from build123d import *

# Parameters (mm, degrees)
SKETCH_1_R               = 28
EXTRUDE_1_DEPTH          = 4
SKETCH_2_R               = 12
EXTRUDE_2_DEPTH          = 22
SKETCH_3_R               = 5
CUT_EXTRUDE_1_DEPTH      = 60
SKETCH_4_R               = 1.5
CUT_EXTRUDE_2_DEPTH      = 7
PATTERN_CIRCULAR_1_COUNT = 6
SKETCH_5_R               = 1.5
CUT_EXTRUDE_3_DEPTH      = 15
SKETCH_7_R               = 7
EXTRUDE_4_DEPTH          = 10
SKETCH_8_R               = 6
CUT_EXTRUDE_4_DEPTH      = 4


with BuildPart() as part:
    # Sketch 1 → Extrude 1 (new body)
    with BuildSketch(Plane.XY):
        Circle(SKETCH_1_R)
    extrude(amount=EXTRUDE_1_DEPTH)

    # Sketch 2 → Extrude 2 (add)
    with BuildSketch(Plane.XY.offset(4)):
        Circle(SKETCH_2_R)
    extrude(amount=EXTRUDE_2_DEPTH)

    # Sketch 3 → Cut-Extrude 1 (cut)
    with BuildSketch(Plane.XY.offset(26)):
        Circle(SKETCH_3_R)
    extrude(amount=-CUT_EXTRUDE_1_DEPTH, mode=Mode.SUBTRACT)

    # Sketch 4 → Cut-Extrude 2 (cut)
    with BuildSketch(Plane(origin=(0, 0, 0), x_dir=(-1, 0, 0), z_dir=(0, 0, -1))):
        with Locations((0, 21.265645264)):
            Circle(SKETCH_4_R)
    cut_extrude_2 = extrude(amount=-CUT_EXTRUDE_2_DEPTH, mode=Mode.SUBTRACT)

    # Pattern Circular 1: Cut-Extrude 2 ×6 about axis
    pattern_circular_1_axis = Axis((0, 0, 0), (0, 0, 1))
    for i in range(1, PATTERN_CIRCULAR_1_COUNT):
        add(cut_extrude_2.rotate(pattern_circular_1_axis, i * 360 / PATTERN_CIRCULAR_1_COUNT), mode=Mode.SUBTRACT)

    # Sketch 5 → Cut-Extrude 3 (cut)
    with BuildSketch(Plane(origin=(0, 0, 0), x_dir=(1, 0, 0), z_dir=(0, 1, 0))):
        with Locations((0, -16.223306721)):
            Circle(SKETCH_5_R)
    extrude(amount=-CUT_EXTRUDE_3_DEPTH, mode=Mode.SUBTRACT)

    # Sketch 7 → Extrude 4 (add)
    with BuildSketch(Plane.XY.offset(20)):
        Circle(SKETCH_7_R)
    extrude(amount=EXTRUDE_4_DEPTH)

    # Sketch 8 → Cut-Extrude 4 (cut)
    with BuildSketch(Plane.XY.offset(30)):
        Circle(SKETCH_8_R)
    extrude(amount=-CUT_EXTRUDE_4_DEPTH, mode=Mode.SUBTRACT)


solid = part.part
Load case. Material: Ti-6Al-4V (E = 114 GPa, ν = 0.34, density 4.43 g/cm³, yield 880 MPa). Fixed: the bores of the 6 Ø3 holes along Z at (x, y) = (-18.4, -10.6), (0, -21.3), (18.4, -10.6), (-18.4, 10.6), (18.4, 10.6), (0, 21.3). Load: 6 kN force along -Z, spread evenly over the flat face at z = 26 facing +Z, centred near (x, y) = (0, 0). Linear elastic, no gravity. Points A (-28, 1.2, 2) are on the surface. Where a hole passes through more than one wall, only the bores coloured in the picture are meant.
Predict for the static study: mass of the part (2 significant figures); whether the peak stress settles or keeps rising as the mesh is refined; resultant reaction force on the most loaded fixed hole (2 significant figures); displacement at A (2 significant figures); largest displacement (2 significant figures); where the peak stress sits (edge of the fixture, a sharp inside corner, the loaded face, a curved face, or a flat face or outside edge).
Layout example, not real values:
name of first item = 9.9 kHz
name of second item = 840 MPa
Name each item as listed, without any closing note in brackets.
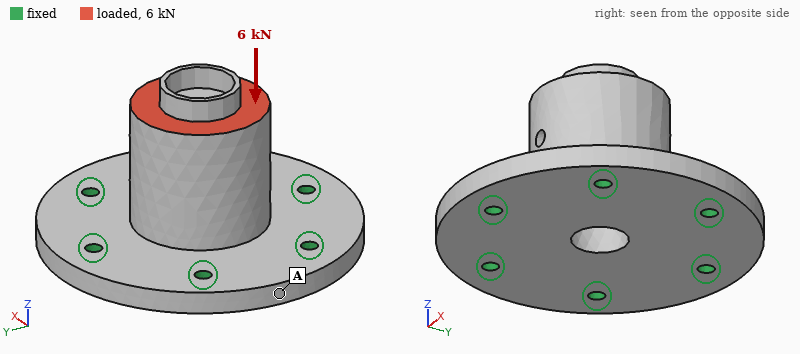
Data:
mass of the part = 81 g
whether the peak stress settles or keeps rising as the mesh is refined = keeps rising
resultant reaction force on the most loaded fixed hole = 1.1 kN
displacement at A = 4.1 µm
largest displacement = 23 µm
where the peak stress sits = edge of the fixture
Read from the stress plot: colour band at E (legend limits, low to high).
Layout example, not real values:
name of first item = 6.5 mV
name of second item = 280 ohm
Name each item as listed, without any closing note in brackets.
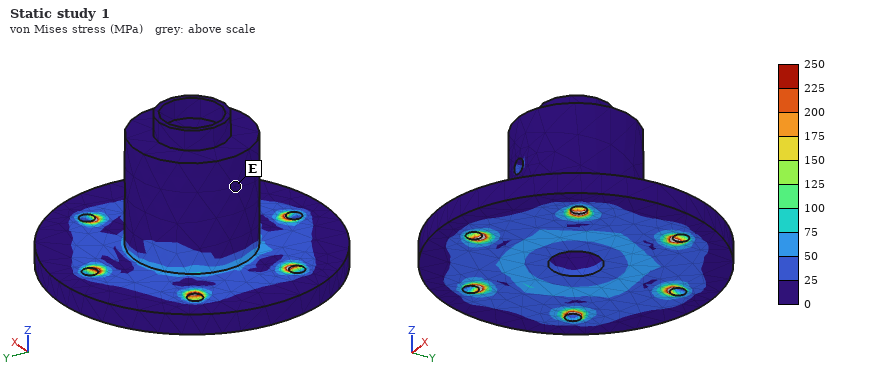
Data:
colour band at E = 0 to 25 MPa
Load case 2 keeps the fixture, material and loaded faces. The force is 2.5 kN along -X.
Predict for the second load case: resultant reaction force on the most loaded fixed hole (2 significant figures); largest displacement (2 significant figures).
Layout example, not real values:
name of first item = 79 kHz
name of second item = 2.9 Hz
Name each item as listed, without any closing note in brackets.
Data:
resultant reaction force on the most loaded fixed hole = 1.1 kN
largest displacement = 48 µm
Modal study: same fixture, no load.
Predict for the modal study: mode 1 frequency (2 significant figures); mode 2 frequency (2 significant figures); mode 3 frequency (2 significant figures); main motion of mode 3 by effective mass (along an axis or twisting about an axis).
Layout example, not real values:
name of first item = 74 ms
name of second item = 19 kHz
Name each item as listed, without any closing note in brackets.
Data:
mode 1 frequency = 9300 Hz
mode 2 frequency = 9300 Hz
mode 3 frequency = 12 kHz
main motion of mode 3 by effective mass = along Z
